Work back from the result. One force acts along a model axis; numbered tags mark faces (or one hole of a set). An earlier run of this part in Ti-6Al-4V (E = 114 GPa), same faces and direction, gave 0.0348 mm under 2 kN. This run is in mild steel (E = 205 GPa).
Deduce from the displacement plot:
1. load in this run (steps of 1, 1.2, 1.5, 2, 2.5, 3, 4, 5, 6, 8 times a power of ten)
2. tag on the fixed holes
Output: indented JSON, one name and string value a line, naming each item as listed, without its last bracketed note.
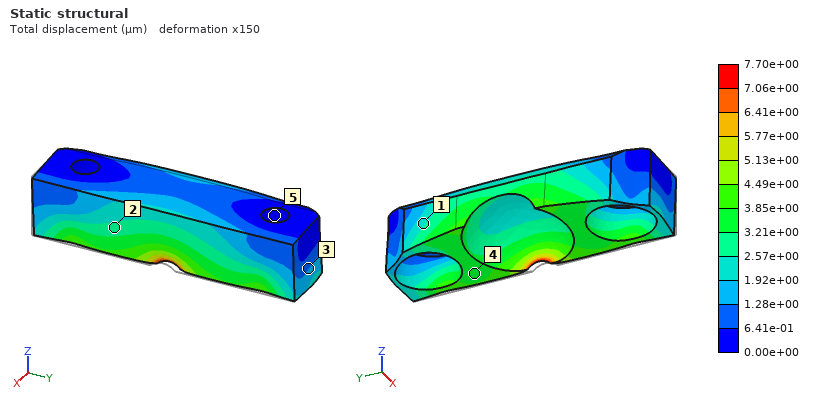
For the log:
{
  "load in this run": "800 N",
  "tag on the fixed holes": "5"
}
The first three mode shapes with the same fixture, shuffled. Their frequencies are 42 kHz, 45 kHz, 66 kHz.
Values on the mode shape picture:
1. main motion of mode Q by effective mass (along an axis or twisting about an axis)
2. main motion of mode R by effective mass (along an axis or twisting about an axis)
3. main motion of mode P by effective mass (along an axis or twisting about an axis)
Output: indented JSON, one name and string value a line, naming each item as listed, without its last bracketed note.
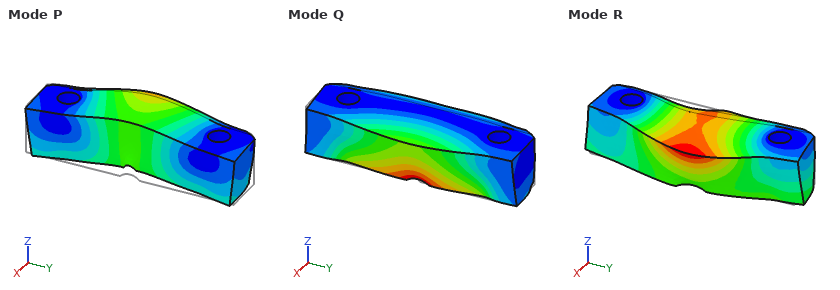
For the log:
{
  "main motion of mode Q by effective mass": "along X",
  "main motion of mode R by effective mass": "along X",
  "main motion of mode P by effective mass": "along Z"
}
